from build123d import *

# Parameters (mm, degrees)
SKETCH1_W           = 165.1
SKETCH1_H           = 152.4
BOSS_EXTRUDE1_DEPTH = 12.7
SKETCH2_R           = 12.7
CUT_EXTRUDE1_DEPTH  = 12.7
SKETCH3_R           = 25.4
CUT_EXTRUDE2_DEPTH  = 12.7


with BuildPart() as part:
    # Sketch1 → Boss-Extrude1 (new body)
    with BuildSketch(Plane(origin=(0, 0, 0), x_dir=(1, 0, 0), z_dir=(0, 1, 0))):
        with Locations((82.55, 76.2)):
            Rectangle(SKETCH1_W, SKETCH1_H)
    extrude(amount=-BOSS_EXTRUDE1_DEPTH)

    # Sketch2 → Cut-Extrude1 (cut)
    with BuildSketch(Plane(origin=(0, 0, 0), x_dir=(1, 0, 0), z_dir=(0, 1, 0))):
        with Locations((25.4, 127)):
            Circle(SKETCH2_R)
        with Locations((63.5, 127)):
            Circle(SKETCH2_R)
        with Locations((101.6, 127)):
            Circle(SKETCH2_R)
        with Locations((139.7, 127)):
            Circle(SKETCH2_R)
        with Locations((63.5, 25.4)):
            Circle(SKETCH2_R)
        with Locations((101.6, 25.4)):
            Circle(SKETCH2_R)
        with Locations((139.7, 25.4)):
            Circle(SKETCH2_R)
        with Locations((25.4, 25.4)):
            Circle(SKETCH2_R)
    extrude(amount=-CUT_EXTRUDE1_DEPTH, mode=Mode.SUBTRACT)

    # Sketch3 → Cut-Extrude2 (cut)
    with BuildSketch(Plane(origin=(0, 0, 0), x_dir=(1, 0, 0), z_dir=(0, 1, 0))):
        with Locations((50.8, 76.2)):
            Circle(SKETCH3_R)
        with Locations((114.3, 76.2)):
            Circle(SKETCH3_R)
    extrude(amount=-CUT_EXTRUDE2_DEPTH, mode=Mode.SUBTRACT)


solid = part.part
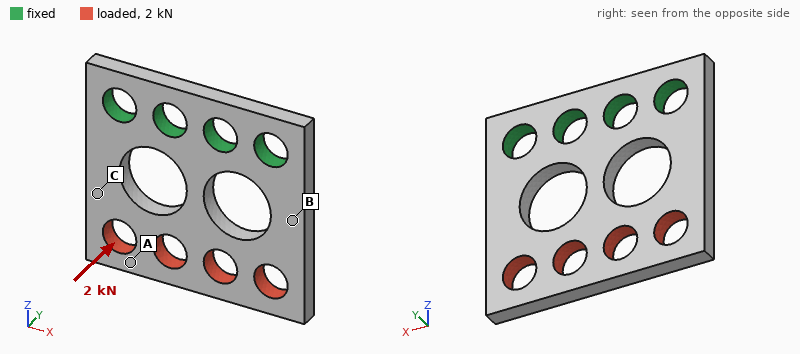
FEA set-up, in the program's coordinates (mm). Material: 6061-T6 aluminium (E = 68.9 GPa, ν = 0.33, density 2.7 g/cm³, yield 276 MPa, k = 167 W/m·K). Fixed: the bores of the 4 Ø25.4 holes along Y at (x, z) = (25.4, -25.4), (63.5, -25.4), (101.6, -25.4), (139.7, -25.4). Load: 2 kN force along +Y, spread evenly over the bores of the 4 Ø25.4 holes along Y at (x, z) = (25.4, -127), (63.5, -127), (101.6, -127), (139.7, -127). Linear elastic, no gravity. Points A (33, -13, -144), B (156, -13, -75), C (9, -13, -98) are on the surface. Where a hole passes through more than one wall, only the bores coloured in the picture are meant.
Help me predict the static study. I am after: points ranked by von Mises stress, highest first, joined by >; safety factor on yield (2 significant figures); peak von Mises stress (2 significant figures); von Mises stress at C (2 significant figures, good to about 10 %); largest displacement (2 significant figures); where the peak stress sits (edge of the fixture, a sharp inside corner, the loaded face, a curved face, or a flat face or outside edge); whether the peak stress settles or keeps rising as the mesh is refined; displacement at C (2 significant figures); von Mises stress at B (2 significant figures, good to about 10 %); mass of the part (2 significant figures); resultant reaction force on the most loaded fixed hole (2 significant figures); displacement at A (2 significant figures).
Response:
B > C > A
2.9
96 MPa
27 MPa
0.73 mm
a curved face
settles
0.25 mm
52 MPa
580 g
700 N
0.64 mm
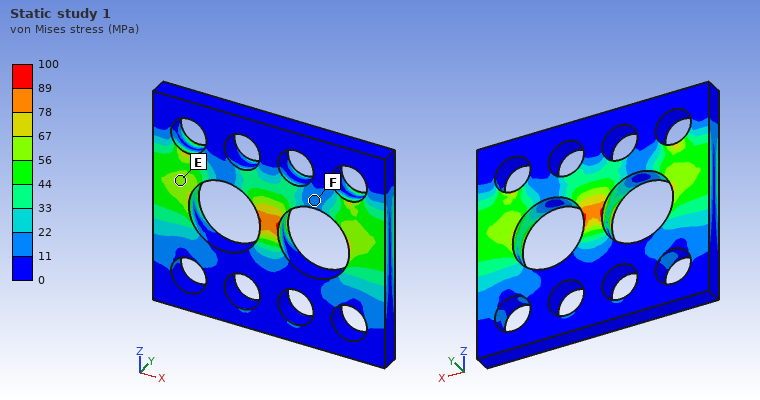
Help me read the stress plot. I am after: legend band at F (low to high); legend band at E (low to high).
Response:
11 to 22 MPa
56 to 67 MPa
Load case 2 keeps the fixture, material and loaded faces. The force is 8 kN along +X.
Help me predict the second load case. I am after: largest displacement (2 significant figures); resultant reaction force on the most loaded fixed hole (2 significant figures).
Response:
96 µm
4.8 kN
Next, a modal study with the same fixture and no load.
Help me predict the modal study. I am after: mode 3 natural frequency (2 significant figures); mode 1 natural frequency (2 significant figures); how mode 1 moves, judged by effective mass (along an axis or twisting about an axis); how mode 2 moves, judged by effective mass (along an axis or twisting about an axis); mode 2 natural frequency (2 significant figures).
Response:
2700 Hz
640 Hz
along Y
twisting about Z
1200 Hz
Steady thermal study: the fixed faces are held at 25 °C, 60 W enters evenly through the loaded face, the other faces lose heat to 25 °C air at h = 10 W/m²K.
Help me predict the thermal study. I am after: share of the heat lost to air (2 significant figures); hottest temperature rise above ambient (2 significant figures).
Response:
10 %
31 K
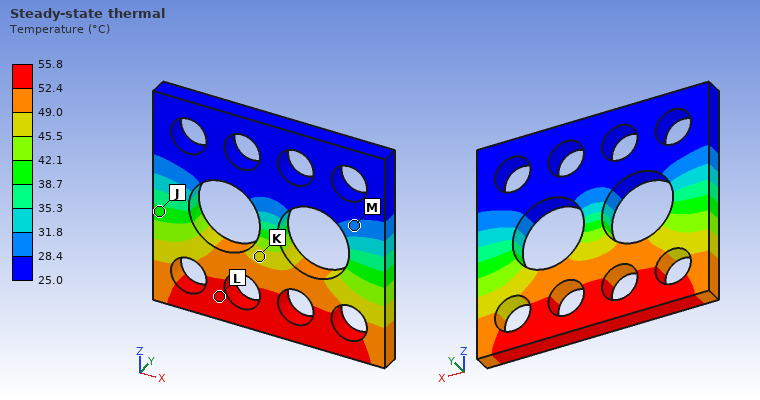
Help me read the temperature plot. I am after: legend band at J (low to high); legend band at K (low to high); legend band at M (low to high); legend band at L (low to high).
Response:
38.7 to 42.1 °C
45.5 to 49.0 °C
28.4 to 31.8 °C
52.4 to 55.8 °C
